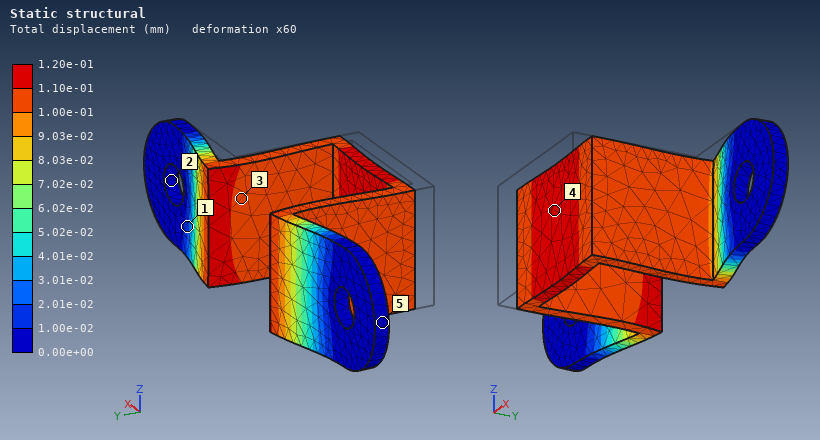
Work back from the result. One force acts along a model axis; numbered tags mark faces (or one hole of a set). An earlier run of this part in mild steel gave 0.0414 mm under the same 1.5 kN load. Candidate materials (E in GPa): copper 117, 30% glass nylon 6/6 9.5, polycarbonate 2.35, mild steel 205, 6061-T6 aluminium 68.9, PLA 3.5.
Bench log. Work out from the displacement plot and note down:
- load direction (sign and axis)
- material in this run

+Y
6061-T6 aluminium
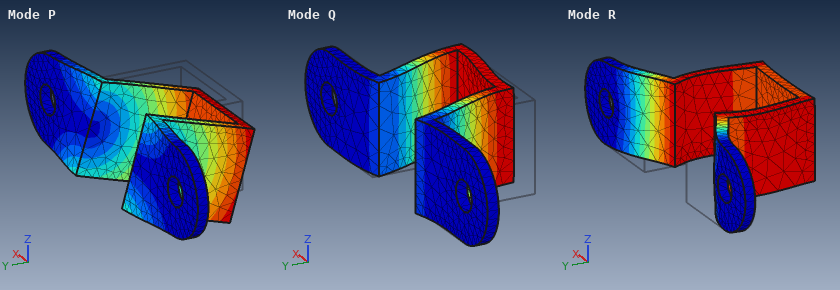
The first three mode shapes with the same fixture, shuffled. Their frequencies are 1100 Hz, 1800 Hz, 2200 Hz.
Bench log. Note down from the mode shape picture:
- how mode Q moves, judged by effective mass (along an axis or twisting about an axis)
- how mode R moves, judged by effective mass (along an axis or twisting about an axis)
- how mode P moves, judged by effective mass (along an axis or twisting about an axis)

along X
along Y
along Z
